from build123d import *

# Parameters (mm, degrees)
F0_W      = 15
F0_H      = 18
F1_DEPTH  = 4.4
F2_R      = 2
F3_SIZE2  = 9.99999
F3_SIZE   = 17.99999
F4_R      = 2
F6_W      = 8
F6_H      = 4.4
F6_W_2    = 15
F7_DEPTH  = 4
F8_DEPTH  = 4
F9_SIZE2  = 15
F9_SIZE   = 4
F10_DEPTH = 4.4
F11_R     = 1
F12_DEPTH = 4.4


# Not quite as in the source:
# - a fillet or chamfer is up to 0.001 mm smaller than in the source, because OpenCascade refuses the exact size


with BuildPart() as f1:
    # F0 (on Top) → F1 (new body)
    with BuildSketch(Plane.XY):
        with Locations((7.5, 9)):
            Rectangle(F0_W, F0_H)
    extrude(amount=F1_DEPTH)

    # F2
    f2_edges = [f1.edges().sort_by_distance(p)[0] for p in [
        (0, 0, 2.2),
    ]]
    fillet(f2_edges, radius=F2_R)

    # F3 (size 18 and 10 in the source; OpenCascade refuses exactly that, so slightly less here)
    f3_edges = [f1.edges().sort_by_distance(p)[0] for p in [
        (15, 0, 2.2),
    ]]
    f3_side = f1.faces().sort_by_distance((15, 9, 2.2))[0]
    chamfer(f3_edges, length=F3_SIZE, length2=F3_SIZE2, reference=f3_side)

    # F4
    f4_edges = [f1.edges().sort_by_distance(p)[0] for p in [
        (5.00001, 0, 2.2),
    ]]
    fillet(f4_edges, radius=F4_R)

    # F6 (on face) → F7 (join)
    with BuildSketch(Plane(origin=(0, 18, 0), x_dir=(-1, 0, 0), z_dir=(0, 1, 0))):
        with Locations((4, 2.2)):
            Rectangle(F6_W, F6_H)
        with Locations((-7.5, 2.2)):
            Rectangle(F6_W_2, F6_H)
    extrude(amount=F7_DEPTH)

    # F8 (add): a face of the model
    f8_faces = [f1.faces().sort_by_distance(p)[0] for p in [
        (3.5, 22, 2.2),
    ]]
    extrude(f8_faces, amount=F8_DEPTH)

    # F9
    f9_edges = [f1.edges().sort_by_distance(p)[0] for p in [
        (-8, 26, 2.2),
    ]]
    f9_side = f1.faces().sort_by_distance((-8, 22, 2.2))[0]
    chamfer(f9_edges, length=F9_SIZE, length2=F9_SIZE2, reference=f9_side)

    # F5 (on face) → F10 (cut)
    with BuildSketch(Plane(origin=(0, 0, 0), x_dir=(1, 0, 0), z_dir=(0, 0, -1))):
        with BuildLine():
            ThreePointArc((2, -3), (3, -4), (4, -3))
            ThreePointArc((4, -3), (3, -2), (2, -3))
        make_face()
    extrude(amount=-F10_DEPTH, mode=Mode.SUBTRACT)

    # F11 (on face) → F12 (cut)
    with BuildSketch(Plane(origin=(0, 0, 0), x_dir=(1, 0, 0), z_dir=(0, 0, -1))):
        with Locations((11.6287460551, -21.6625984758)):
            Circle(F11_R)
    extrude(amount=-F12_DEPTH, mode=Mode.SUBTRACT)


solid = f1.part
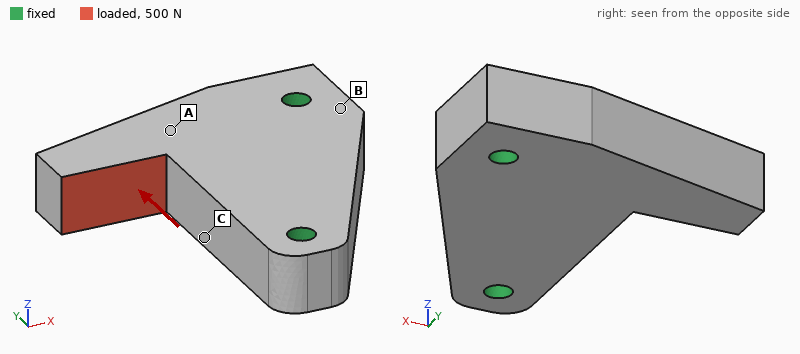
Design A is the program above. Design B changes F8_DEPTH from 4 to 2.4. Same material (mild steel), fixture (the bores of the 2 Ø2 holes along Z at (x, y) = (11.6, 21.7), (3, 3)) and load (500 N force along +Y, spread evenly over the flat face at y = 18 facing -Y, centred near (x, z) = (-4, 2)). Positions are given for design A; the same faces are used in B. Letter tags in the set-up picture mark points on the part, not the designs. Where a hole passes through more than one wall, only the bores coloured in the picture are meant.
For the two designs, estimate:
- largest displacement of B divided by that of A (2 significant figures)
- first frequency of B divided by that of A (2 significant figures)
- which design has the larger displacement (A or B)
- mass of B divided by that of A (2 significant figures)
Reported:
1.7
1.1
B
0.89
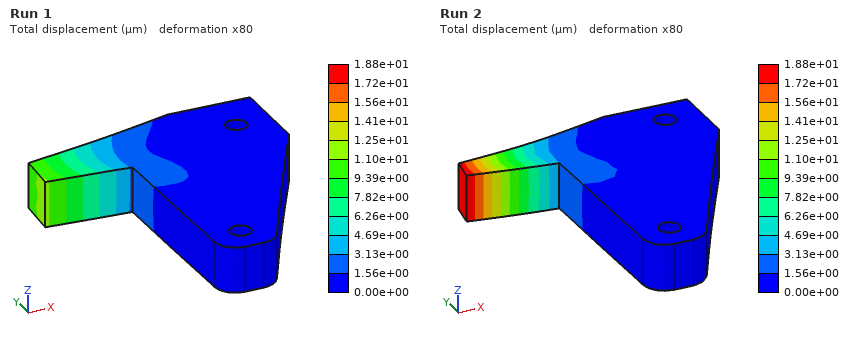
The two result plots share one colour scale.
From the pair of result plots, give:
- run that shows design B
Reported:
Run 2
